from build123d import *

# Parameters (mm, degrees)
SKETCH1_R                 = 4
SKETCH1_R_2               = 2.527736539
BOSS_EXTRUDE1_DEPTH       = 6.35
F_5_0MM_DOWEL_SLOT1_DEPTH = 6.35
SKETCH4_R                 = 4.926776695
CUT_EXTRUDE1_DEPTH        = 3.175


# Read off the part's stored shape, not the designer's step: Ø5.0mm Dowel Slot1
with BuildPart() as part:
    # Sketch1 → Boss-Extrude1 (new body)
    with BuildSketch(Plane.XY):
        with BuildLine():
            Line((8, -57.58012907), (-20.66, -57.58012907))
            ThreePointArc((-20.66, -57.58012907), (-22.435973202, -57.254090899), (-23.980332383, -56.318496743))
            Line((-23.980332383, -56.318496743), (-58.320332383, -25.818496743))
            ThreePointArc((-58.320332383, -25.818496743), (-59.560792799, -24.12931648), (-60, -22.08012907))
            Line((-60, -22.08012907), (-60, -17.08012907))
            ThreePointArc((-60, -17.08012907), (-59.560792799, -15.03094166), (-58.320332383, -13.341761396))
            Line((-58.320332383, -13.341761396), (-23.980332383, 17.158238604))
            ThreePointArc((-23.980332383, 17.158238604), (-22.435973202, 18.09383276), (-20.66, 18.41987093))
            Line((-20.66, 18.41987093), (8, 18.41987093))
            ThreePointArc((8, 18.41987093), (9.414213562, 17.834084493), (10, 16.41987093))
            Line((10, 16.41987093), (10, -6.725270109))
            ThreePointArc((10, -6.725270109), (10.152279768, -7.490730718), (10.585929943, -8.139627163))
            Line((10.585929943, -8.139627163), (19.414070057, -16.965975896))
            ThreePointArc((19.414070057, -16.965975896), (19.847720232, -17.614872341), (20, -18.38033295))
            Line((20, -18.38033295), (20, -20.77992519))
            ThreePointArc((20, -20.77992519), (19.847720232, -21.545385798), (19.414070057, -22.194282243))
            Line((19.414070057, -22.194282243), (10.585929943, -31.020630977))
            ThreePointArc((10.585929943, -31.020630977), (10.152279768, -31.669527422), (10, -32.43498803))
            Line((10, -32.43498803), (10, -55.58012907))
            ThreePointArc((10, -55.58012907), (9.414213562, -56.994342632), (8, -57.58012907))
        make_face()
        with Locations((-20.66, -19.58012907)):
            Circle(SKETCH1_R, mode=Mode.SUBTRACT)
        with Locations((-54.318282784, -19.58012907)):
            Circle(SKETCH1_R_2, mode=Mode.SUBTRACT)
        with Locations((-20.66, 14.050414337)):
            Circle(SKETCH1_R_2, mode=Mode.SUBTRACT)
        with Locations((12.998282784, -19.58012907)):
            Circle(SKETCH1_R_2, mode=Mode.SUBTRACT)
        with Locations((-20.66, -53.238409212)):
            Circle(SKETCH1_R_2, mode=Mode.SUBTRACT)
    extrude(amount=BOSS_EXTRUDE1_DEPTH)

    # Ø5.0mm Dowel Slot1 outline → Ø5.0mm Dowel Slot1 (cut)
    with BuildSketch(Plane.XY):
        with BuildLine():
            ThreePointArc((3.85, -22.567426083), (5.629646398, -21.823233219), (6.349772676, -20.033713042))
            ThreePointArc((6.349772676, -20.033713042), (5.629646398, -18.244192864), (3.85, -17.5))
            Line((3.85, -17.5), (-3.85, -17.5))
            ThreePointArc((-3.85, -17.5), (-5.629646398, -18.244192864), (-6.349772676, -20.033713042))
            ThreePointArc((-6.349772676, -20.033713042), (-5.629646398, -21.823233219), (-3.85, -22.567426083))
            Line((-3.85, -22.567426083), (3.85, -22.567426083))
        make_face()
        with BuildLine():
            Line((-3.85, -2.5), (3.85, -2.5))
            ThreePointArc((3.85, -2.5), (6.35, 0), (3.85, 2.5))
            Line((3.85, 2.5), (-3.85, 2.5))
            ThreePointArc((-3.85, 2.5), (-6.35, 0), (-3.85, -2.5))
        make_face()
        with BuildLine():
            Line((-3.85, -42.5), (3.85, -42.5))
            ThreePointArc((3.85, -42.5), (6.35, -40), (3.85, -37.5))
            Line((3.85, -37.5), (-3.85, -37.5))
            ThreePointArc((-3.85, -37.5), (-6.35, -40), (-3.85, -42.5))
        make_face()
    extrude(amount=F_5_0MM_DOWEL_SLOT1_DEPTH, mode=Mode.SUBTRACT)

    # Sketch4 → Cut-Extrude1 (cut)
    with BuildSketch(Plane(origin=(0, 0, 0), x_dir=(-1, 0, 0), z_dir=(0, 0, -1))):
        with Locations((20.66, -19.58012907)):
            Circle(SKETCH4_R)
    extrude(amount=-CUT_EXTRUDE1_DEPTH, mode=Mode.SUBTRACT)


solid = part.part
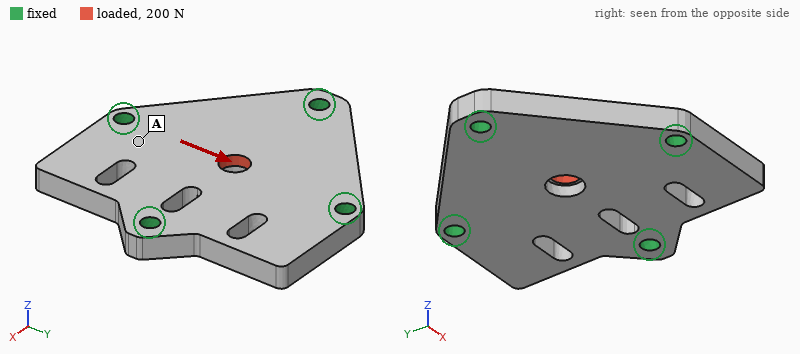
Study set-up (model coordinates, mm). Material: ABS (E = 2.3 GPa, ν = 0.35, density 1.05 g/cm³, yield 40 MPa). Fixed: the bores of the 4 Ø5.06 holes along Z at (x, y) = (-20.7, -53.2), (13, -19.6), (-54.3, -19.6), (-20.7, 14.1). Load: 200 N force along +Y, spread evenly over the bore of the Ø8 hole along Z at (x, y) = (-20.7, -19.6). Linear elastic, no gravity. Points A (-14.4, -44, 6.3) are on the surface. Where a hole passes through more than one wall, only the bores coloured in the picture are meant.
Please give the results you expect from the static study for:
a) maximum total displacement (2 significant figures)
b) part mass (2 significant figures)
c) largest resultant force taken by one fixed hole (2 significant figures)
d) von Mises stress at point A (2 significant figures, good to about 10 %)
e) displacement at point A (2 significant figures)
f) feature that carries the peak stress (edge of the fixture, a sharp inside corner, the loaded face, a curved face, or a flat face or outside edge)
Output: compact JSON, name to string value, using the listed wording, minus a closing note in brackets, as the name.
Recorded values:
{"maximum total displacement": "15 µm", "part mass": "26 g", "largest resultant force taken by one fixed hole": "76 N", "von Mises stress at point A": "0.58 MPa", "displacement at point A": "3.5 µm", "feature that carries the peak stress": "a sharp inside corner"}
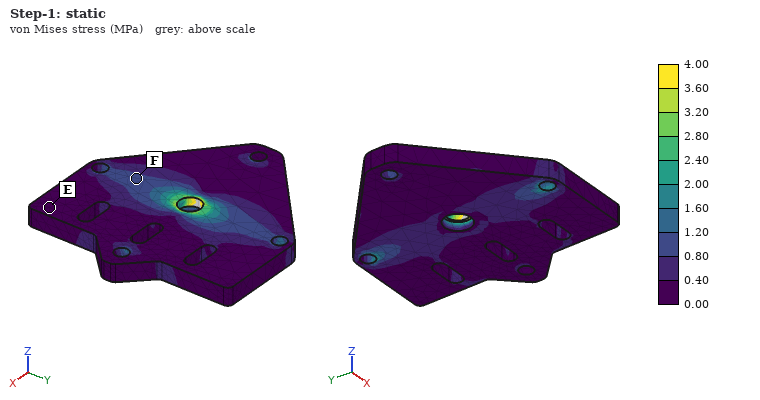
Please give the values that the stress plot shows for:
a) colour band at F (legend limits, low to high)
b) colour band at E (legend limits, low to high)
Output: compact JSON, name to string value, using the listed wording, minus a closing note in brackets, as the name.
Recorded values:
{"colour band at F": "0.80 to 1.20 MPa", "colour band at E": "0.00 to 0.40 MPa"}
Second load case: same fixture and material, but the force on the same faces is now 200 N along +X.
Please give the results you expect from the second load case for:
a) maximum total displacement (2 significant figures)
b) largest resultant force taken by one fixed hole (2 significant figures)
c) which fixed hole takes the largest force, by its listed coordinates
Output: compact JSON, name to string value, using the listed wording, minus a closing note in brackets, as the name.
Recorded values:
{"maximum total displacement": "17 µm", "largest resultant force taken by one fixed hole": "83 N", "which fixed hole takes the largest force, by its listed coordinates": "(-54.3, -19.6)"}
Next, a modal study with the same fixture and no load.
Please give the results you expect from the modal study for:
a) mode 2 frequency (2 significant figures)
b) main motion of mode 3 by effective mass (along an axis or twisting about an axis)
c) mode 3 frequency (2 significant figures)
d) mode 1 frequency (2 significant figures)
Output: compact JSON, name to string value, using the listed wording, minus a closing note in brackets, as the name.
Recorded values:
{"mode 2 frequency": "2500 Hz", "main motion of mode 3 by effective mass": "along Z", "mode 3 frequency": "2800 Hz", "mode 1 frequency": "2500 Hz"}
